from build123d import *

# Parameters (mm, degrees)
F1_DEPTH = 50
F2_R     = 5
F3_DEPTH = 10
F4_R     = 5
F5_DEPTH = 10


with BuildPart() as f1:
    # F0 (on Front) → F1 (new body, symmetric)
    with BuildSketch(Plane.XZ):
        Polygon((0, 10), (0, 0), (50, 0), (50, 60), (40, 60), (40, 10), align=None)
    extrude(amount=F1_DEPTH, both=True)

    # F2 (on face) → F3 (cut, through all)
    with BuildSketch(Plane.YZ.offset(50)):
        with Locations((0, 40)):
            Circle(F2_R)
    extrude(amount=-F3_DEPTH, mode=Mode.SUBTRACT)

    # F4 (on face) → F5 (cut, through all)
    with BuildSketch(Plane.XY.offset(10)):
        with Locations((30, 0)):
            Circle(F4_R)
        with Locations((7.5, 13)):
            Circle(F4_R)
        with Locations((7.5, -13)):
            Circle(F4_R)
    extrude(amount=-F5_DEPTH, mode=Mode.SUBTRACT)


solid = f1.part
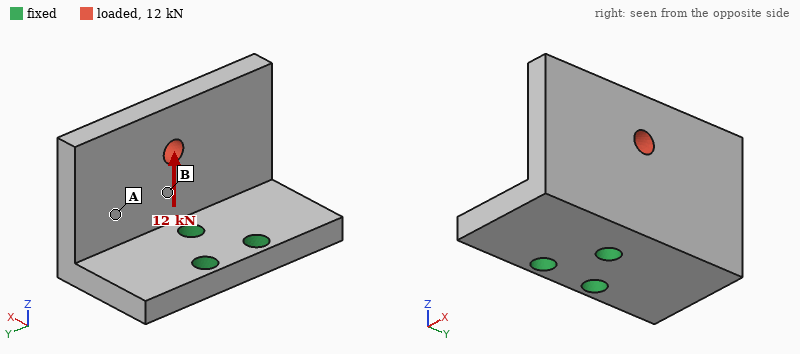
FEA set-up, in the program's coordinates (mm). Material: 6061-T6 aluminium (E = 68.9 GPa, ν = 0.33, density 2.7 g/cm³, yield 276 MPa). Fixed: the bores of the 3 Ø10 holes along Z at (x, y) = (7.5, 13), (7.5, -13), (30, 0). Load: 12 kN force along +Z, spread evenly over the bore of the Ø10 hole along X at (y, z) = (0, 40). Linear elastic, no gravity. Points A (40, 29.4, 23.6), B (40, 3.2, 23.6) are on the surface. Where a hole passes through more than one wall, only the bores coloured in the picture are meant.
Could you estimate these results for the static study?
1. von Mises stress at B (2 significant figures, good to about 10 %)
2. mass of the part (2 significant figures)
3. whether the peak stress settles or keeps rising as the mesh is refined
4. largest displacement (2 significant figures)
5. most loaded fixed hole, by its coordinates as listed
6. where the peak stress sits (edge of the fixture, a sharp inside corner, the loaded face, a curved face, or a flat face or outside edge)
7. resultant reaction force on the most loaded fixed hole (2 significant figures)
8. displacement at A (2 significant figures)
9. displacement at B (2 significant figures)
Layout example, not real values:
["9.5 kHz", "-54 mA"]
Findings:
["44 MPa", "260 g", "keeps rising", "0.21 mm", "(30, 0)", "edge of the fixture", "14 kN", "0.076 mm", "0.081 mm"]
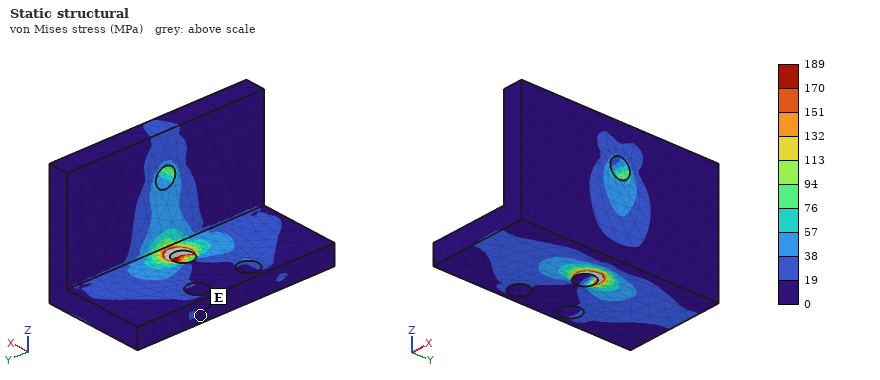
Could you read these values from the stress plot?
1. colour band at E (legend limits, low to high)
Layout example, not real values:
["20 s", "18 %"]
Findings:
["0 to 19 MPa"]
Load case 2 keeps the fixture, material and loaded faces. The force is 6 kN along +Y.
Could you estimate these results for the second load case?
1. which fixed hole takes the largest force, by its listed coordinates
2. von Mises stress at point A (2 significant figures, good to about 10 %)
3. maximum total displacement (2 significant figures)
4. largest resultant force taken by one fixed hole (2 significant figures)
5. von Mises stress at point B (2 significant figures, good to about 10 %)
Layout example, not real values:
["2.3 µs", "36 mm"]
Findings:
["(30, 0)", "30 MPa", "0.31 mm", "6.7 kN", "42 MPa"]
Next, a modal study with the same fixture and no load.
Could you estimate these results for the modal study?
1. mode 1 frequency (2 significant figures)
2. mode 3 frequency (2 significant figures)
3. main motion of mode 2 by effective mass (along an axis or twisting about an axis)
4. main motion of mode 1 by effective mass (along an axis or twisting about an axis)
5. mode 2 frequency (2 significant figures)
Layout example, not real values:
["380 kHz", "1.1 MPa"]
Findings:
["1800 Hz", "3500 Hz", "along Y", "along X", "2000 Hz"]
